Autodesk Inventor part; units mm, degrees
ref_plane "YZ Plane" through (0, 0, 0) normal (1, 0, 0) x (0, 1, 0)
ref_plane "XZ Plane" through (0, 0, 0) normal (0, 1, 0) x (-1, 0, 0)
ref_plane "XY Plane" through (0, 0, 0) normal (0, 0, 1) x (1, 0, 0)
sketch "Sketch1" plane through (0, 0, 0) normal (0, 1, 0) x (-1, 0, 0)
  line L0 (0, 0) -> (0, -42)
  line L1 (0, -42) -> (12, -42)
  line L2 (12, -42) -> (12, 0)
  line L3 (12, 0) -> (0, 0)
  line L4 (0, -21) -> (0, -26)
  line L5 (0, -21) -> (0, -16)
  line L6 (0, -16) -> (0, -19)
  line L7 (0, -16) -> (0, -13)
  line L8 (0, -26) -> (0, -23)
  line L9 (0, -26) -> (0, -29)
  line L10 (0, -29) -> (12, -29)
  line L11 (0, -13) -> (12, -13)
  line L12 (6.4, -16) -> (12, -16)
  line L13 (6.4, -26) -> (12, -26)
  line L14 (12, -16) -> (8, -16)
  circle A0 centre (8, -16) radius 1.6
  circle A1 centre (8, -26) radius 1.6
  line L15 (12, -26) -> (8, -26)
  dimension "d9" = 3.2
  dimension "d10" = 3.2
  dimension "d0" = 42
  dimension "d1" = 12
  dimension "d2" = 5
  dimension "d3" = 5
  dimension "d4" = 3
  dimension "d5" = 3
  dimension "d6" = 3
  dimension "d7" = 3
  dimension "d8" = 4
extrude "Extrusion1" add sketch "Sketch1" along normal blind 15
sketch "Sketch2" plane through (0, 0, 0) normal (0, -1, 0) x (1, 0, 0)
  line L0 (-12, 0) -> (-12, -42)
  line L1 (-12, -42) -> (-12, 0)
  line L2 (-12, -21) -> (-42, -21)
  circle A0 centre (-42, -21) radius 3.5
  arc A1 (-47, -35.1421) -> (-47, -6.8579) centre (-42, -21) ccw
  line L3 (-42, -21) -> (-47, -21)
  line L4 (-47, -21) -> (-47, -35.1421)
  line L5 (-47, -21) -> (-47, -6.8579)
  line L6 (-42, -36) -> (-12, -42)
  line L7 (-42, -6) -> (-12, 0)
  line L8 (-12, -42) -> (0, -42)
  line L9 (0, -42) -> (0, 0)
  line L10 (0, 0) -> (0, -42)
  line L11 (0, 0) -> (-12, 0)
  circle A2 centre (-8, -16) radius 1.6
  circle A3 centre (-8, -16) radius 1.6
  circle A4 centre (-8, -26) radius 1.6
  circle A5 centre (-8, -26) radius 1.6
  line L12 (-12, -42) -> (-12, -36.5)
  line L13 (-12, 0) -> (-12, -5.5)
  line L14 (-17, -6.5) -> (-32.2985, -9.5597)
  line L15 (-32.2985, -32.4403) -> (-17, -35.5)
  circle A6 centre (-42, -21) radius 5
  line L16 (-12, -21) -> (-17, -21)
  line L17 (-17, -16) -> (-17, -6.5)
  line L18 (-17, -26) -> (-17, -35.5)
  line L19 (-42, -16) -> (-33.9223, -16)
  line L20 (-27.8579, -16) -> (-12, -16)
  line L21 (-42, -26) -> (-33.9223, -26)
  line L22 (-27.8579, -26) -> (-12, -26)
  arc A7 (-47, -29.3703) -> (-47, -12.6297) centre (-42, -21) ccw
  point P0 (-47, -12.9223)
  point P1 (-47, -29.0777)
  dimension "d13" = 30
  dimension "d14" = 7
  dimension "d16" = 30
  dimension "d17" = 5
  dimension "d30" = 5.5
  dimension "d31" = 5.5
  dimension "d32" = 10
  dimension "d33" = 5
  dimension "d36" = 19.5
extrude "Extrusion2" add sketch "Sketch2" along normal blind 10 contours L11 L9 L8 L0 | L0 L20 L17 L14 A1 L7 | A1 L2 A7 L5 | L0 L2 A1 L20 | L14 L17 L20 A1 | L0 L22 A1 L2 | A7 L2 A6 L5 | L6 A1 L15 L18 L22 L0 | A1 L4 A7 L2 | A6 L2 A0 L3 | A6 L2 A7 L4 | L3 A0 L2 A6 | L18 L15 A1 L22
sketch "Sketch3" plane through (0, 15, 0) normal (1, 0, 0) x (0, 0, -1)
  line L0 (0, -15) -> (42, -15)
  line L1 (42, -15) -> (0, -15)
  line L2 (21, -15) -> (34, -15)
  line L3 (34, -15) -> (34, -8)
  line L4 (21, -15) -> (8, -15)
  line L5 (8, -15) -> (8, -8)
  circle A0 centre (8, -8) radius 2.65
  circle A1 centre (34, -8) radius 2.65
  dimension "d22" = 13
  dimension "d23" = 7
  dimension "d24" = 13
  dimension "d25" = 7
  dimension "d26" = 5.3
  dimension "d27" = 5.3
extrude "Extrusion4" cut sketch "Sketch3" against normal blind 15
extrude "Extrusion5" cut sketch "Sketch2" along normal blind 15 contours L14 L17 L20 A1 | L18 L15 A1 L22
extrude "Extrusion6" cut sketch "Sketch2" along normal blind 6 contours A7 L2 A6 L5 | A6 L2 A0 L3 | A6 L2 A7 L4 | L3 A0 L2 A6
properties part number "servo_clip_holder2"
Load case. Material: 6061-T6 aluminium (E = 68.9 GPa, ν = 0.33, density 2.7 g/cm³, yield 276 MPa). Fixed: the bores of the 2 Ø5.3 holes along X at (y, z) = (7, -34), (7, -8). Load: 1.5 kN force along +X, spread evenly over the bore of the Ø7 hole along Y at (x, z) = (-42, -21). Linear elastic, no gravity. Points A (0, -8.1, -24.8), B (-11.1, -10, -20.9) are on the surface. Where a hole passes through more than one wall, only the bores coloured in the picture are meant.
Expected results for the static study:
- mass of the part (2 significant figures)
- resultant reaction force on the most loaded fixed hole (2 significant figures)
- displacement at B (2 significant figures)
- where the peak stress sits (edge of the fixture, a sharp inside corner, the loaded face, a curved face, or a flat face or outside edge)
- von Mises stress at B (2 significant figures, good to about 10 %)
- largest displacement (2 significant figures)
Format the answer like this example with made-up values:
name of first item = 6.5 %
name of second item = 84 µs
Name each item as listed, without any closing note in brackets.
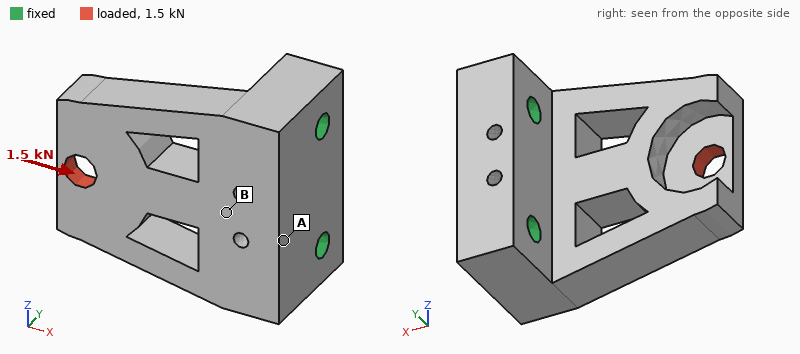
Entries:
mass of the part = 55 g
resultant reaction force on the most loaded fixed hole = 750 N
displacement at B = 9.3 µm
where the peak stress sits = a flat face or outside edge
von Mises stress at B = 16 MPa
largest displacement = 50 µm
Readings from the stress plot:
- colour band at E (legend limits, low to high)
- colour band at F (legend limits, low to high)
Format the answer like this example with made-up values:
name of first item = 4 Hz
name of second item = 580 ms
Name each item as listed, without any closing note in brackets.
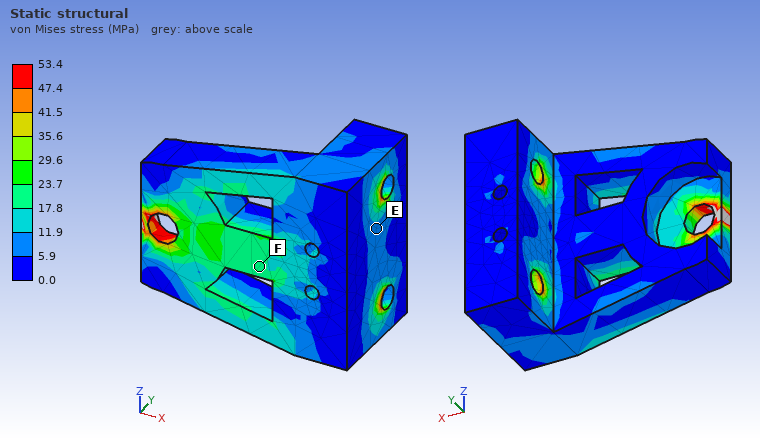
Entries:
colour band at E = 5.9 to 11.9 MPa
colour band at F = 17.8 to 23.7 MPa
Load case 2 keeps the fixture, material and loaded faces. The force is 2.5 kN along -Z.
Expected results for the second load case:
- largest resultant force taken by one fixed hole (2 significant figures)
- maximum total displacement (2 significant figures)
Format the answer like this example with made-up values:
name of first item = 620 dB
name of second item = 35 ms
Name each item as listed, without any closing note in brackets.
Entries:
largest resultant force taken by one fixed hole = 3.2 kN
maximum total displacement = 72 µm
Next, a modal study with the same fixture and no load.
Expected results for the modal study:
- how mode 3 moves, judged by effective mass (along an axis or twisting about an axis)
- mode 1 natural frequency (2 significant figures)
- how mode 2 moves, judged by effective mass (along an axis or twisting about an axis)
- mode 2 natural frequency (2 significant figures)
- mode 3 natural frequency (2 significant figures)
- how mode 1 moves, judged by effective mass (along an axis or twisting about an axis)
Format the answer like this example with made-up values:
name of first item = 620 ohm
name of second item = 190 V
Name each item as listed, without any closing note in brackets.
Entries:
how mode 3 moves, judged by effective mass = along Z
mode 1 natural frequency = 4800 Hz
how mode 2 moves, judged by effective mass = along Z
mode 2 natural frequency = 9100 Hz
mode 3 natural frequency = 10 kHz
how mode 1 moves, judged by effective mass = along Y
